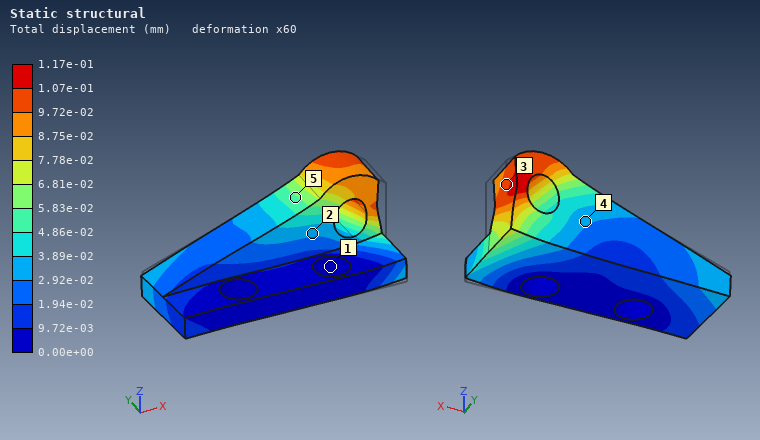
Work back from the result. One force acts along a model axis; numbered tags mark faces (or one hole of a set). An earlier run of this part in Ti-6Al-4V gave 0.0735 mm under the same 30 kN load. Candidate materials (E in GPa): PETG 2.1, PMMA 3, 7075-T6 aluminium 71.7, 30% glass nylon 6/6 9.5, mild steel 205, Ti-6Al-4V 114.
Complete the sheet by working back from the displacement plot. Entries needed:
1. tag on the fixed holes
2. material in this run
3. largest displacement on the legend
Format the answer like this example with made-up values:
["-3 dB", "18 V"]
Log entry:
["1", "7075-T6 aluminium", "1.17e-01 mm"]
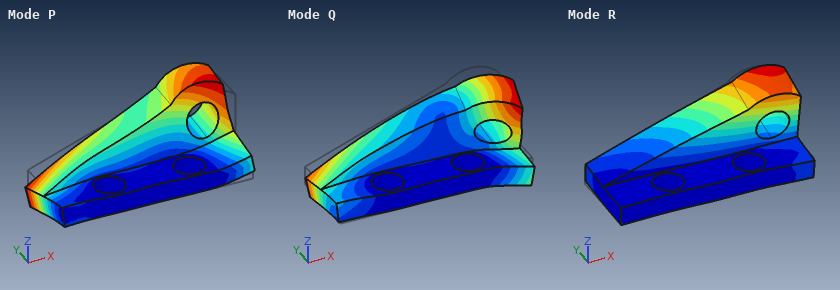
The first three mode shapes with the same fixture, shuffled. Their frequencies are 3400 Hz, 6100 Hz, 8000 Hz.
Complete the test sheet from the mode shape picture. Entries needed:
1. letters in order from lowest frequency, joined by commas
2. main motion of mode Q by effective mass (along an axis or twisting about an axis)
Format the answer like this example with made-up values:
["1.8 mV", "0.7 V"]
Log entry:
["R, P, Q", "along Z"]
